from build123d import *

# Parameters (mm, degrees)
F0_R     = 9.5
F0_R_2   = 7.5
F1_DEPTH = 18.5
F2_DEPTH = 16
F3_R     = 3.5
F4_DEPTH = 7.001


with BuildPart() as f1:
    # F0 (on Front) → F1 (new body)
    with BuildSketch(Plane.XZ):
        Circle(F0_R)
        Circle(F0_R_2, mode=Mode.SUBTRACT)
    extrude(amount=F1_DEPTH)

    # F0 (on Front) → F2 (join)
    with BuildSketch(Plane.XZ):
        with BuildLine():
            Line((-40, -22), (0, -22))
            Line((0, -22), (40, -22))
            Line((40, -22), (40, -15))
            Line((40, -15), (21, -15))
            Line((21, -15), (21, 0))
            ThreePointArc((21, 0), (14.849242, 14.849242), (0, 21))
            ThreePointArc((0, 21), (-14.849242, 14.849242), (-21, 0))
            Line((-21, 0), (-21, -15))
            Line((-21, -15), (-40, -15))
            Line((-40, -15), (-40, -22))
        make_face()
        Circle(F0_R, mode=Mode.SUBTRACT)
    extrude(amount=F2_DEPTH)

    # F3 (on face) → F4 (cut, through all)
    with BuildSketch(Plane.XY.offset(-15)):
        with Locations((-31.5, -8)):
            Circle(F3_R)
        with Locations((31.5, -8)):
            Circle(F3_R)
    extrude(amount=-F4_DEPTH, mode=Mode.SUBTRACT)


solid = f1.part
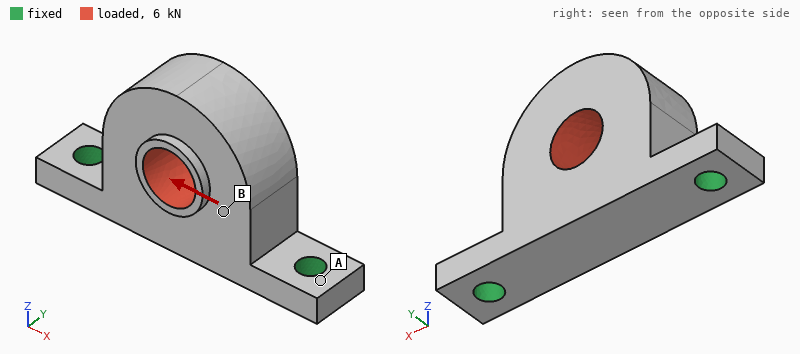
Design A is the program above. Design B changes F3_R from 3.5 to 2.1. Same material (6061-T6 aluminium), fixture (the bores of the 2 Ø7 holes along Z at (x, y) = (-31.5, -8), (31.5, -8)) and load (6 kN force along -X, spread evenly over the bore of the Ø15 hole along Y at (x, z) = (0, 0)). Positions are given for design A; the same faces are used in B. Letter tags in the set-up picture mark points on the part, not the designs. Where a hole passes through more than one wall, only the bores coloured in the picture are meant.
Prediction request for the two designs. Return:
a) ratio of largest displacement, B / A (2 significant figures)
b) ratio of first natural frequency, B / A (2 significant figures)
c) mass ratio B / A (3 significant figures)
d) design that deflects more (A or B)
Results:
1.2
0.89
1.01
B
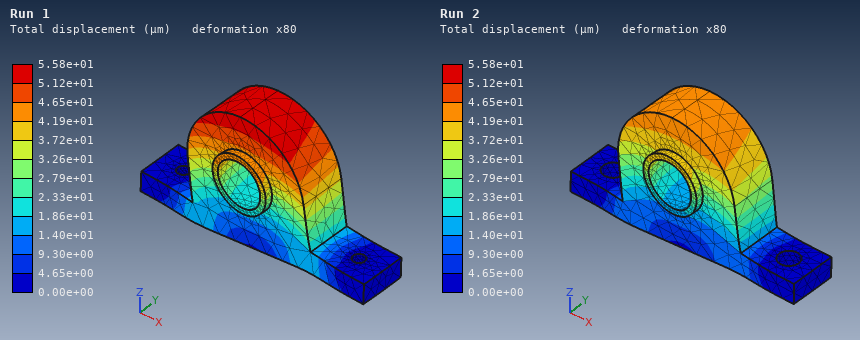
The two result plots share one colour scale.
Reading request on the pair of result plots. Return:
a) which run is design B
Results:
Run 1
